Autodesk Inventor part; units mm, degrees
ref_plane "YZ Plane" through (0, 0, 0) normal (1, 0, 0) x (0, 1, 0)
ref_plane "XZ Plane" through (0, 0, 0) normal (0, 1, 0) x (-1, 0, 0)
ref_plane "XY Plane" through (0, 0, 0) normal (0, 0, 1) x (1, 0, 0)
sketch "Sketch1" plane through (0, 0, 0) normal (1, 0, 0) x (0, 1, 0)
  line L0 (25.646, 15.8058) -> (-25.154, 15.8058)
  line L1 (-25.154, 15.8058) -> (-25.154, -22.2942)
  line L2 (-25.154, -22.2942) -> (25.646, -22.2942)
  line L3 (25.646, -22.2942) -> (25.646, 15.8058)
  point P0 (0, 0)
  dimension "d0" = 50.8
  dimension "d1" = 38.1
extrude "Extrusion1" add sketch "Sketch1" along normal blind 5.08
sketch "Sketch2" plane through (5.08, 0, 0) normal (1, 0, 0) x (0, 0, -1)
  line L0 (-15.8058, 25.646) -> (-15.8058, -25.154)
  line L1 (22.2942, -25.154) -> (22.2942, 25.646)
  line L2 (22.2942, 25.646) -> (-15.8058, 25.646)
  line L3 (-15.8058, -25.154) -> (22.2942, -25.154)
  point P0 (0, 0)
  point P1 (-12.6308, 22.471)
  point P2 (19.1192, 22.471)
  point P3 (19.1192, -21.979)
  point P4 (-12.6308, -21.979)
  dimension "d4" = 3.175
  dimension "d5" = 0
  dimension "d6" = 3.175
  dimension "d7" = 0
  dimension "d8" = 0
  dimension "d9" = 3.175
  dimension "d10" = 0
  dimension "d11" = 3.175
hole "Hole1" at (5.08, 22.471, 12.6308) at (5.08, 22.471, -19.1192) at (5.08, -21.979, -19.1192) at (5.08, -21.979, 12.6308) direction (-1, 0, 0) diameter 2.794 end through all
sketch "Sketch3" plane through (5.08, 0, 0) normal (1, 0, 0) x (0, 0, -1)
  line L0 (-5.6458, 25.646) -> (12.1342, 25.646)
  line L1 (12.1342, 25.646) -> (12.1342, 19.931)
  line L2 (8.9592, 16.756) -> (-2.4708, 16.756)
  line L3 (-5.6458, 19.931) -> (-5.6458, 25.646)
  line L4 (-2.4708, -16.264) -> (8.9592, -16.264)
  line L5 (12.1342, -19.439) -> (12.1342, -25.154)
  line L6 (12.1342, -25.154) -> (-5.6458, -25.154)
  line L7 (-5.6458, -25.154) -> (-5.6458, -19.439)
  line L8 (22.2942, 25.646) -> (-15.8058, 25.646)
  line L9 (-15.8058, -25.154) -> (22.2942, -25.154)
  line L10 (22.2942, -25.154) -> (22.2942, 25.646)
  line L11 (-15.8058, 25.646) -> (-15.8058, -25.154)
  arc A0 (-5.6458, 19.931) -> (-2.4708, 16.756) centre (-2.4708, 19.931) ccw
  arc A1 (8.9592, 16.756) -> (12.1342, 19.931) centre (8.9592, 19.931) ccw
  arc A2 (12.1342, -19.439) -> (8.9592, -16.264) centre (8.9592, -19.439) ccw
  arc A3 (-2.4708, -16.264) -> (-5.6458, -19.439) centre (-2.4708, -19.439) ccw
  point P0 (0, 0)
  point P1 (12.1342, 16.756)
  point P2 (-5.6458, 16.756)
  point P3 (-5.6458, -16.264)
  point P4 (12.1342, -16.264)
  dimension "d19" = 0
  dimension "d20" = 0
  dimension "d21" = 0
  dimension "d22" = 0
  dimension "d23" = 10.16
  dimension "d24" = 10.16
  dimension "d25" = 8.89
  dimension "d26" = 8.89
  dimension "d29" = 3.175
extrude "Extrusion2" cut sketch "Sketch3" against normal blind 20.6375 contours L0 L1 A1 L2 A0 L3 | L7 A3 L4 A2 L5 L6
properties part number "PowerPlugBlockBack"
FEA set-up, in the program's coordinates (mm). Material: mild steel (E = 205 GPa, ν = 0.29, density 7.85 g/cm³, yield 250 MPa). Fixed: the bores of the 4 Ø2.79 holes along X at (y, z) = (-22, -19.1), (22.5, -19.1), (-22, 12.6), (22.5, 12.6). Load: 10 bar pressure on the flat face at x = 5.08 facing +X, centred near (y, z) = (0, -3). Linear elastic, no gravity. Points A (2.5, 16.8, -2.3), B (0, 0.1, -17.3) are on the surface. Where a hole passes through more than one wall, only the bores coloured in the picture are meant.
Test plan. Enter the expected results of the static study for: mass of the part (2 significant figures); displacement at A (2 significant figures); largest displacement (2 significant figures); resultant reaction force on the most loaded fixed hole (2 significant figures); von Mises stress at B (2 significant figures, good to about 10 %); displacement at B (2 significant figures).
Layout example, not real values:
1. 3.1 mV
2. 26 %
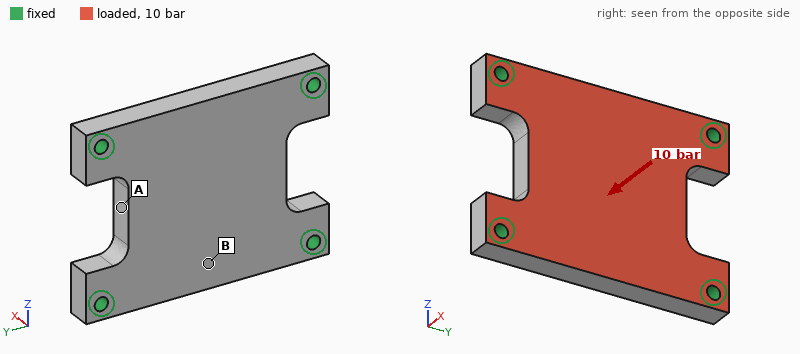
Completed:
1. 64 g
2. 5.0 µm
3. 8.8 µm
4. 400 N
5. 24 MPa
6. 7.7 µm
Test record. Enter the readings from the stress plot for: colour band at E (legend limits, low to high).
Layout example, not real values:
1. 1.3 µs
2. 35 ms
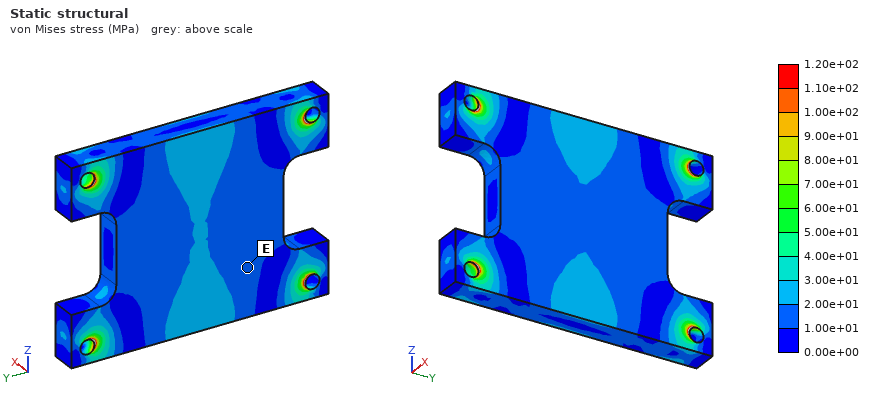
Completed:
1. 1.00e+01 to 2.00e+01 MPa
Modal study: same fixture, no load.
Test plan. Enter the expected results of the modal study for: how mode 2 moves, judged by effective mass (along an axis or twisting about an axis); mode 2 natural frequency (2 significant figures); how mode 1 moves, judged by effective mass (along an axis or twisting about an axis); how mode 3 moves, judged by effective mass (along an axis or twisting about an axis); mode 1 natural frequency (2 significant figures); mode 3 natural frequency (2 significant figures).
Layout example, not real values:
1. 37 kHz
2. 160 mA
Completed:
1. twisting about Y
2. 15 kHz
3. along X
4. twisting about Z
5. 9700 Hz
6. 22 kHz
